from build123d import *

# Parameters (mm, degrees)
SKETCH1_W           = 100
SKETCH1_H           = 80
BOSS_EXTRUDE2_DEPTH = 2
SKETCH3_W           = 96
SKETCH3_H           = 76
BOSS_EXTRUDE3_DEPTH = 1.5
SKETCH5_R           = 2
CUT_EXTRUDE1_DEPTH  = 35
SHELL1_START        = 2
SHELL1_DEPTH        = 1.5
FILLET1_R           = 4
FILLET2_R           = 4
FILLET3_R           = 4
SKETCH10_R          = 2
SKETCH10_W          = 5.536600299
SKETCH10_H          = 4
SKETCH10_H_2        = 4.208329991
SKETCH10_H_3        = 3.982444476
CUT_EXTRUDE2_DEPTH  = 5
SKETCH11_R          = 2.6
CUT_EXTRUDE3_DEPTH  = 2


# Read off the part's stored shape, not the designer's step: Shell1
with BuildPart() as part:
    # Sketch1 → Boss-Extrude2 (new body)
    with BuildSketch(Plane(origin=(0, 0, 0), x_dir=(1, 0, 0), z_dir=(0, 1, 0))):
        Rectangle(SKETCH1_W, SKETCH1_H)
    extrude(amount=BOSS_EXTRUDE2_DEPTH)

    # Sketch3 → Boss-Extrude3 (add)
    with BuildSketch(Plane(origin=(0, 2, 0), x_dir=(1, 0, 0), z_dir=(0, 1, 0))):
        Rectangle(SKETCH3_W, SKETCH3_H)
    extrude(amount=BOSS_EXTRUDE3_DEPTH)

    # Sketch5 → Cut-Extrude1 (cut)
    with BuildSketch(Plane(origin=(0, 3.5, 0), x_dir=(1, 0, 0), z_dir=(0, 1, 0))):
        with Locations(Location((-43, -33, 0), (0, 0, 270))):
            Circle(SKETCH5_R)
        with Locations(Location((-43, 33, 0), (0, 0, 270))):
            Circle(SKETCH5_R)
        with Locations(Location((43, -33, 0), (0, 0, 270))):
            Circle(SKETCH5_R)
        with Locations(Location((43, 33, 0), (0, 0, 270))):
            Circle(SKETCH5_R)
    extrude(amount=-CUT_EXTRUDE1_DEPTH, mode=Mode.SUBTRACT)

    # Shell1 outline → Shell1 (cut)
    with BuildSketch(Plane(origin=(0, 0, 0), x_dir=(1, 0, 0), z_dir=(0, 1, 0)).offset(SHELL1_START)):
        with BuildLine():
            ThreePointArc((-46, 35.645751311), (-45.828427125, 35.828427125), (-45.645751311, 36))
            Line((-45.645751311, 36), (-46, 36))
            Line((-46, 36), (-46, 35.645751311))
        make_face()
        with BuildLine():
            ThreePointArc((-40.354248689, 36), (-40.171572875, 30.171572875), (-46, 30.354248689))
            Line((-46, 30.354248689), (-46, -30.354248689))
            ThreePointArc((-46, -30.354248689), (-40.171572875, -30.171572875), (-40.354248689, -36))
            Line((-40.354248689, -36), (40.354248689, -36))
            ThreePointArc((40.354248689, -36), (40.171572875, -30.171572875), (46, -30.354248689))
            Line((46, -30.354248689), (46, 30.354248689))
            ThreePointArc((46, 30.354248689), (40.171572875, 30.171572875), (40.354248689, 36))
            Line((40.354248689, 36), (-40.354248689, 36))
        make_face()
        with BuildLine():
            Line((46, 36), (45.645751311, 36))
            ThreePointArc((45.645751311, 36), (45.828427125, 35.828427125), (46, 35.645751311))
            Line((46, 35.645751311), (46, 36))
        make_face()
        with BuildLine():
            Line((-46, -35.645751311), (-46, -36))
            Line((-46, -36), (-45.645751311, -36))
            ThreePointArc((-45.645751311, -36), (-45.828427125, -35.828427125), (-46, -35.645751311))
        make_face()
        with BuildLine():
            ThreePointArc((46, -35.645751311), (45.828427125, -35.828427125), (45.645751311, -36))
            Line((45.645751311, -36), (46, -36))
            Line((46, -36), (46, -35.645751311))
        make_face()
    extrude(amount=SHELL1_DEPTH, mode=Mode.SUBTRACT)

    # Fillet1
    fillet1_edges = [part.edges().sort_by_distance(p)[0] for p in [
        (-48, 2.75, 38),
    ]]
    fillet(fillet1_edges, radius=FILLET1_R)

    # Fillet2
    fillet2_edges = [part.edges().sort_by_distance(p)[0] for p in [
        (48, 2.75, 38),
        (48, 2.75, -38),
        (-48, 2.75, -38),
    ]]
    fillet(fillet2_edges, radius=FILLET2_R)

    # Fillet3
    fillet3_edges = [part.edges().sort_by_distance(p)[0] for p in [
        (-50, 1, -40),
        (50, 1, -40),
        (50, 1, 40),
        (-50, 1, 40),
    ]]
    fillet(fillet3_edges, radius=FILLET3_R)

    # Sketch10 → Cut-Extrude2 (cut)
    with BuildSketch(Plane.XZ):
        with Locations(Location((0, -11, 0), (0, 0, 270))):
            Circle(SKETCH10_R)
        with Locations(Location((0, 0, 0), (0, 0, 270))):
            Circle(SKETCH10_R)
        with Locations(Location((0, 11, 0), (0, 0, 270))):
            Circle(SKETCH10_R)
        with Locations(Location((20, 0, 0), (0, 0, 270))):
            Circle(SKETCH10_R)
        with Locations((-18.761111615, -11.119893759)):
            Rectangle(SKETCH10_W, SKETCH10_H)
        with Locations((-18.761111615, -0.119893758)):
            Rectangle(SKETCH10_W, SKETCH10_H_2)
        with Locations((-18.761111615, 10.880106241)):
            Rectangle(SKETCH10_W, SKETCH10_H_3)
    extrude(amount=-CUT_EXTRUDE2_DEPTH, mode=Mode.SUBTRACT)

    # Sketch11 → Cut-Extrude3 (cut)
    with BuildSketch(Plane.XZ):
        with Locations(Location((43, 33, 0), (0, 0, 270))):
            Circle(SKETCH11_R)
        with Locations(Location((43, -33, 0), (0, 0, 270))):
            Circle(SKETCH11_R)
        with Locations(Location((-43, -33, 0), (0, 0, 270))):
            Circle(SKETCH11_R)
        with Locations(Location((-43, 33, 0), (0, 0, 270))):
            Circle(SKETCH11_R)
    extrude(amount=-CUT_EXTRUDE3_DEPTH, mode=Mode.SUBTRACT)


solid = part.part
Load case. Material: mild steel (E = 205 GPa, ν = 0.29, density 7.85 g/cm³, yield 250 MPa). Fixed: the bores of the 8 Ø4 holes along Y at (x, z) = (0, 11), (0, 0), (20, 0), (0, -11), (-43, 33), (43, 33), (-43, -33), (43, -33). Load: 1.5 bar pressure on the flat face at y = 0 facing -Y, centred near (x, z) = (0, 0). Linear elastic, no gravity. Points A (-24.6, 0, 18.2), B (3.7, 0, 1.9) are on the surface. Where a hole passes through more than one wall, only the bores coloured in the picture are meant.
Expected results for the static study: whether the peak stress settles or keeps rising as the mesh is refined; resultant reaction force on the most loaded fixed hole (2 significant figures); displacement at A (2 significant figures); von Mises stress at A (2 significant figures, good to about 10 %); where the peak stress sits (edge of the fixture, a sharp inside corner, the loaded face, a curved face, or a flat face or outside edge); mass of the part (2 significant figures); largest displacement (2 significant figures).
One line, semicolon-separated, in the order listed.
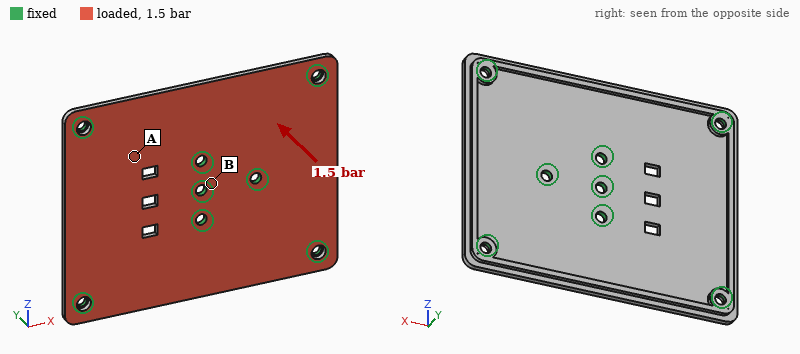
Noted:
keeps rising; 280 N; 20 µm; 27 MPa; edge of the fixture; 130 g; 39 µm
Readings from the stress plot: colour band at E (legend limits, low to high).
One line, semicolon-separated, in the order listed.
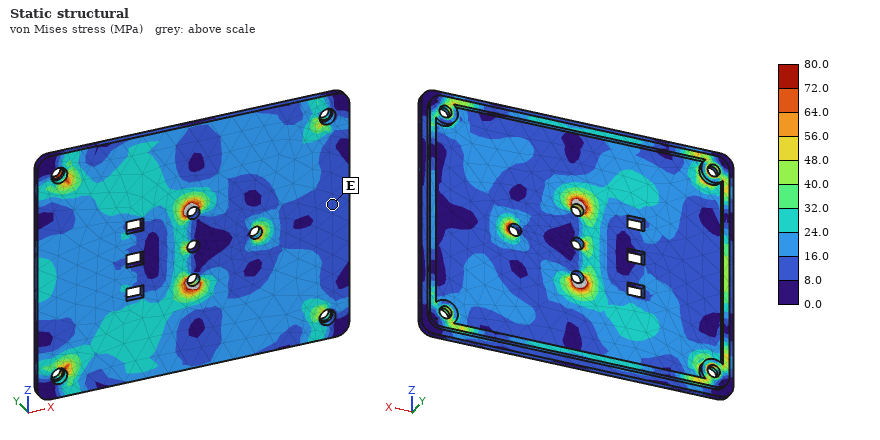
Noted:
8.0 to 16.0 MPa
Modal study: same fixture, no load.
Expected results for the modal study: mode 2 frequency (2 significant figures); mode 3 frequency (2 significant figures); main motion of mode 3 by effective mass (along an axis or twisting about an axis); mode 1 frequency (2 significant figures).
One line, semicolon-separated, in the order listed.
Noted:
3000 Hz; 3200 Hz; along Y; 2900 Hz
